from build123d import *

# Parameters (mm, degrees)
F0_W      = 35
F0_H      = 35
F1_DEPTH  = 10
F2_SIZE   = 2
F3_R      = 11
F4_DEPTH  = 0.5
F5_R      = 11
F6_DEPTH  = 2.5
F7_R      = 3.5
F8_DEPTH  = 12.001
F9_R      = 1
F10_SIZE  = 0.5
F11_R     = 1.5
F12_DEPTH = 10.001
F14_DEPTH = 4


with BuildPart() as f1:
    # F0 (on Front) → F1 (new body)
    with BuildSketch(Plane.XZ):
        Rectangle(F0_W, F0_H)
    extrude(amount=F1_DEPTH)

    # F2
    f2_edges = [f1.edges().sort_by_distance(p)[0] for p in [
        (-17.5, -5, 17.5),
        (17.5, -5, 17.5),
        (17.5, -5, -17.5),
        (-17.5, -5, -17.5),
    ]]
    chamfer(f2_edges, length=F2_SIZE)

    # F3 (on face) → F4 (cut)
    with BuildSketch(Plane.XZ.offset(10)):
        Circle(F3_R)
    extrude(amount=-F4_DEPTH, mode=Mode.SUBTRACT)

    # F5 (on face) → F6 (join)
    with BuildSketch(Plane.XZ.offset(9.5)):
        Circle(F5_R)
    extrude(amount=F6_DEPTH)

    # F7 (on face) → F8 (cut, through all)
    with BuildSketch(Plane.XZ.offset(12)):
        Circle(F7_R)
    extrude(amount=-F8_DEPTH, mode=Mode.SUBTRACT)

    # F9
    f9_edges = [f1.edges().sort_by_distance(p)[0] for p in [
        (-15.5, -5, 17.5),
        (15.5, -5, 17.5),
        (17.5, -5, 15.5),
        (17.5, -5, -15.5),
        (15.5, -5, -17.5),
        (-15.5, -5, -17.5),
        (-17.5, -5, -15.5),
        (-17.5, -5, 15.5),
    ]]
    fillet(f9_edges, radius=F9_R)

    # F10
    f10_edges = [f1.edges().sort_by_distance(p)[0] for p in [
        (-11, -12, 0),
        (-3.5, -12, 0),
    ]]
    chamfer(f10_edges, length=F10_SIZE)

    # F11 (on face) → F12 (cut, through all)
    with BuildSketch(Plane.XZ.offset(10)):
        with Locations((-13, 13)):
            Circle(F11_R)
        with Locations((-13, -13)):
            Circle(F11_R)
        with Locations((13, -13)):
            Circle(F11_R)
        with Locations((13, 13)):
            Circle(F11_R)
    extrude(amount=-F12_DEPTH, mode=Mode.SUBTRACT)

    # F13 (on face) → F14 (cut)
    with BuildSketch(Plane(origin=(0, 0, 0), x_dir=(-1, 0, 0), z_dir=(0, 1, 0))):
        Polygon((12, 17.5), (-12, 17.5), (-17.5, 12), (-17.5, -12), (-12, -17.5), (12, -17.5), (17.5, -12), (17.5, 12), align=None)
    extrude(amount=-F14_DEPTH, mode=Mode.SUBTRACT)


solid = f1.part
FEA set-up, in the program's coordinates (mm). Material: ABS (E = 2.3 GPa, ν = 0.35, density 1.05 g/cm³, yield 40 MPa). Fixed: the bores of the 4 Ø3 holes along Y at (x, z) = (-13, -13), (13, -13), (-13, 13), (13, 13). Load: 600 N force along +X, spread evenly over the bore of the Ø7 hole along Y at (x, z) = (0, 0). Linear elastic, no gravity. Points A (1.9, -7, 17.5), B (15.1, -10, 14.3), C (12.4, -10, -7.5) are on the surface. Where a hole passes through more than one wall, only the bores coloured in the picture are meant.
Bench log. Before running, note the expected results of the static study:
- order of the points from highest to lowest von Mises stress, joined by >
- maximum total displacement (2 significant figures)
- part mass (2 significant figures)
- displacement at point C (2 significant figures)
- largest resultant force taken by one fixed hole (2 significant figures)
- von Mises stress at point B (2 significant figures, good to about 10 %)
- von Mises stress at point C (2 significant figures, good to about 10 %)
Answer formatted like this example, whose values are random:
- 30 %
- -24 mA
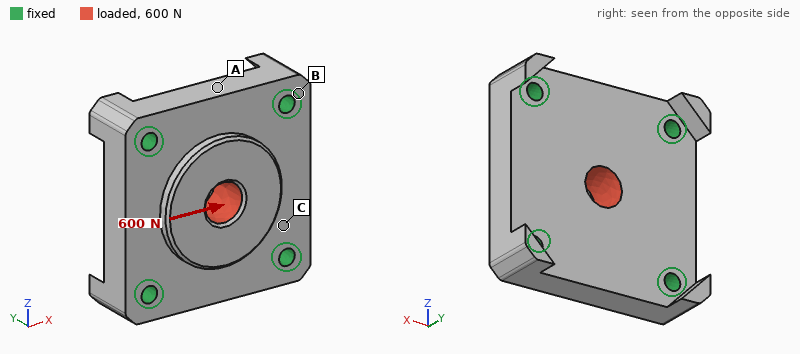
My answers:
- C > B > A
- 27 µm
- 8.2 g
- 12 µm
- 170 N
- 1.3 MPa
- 2.5 MPa
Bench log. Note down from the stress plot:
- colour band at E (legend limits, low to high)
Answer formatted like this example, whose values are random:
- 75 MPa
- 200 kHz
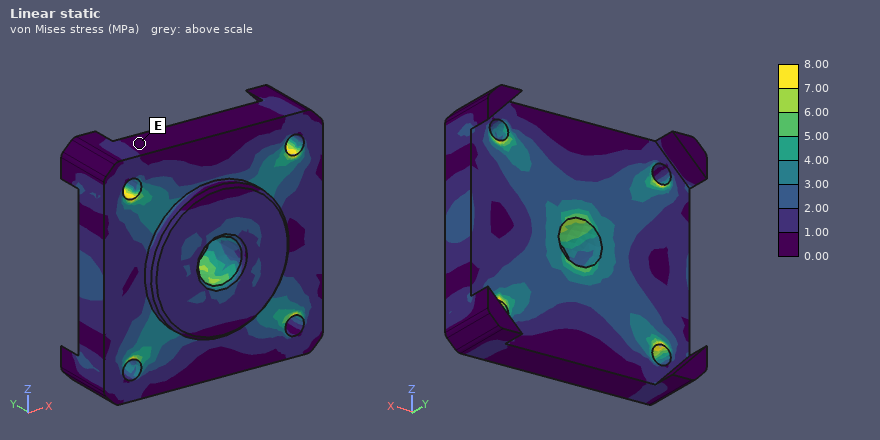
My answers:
- 0.00 to 1.00 MPa
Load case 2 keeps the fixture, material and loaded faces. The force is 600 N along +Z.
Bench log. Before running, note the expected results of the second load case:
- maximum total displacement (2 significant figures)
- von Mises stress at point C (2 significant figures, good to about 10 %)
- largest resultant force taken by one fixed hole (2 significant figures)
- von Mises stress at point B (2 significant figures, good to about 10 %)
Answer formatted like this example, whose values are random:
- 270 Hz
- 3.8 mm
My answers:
- 27 µm
- 2.6 MPa
- 170 N
- 1.2 MPa
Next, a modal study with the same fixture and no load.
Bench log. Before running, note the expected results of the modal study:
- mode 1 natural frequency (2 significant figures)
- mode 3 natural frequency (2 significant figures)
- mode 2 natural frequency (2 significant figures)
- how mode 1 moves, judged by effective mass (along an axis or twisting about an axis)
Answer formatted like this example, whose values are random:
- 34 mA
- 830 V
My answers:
- 7800 Hz
- 11 kHz
- 11 kHz
- along Y
